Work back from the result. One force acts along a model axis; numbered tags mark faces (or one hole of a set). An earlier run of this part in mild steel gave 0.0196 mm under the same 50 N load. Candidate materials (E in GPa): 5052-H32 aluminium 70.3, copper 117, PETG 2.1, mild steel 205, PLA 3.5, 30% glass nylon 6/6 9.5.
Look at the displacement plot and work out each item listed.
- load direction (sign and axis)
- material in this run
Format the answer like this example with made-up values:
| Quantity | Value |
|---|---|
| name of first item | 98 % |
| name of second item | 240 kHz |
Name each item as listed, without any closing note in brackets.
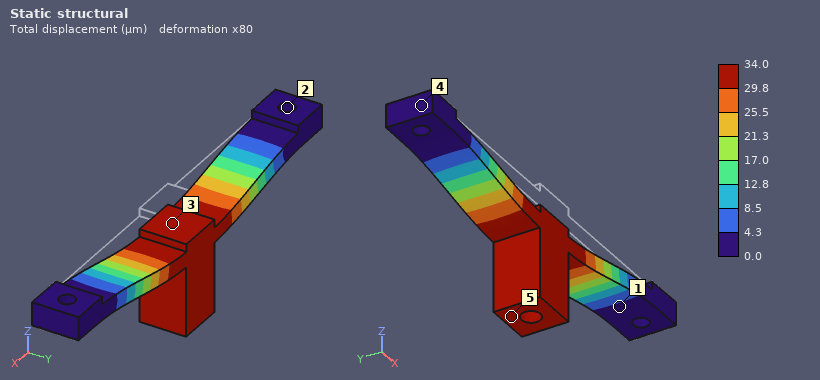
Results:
| Quantity | Value |
|---|---|
| load direction | -Z |
| material in this run | copper |
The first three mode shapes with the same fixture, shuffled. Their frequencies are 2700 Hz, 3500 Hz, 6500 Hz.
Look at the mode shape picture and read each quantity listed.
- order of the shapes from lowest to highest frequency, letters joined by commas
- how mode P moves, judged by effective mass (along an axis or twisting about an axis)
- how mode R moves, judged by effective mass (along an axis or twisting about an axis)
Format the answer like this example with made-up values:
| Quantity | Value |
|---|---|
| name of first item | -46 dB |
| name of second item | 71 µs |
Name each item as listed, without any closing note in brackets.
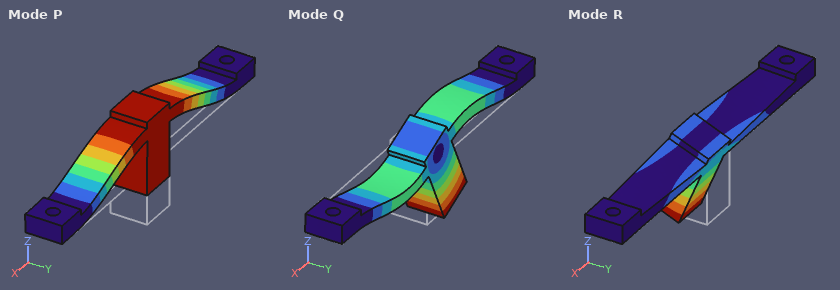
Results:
| Quantity | Value |
|---|---|
| order of the shapes from lowest to highest frequency, letters joined by commas | P, R, Q |
| how mode P moves, judged by effective mass | along Z |
| how mode R moves, judged by effective mass | along Y |
